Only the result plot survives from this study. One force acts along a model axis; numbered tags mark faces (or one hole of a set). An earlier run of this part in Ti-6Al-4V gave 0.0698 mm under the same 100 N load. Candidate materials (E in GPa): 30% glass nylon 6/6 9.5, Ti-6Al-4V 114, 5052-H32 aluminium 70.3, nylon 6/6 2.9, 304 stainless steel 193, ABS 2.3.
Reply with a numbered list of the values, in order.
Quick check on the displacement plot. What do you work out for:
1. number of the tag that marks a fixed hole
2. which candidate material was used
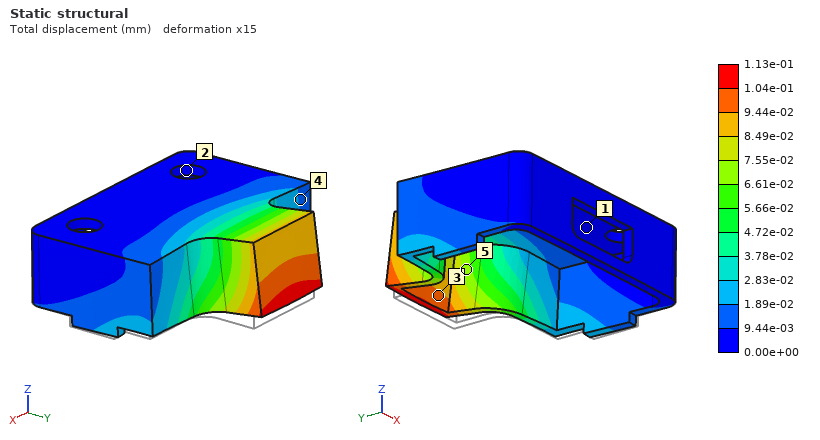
1. 2
2. 5052-H32 aluminium
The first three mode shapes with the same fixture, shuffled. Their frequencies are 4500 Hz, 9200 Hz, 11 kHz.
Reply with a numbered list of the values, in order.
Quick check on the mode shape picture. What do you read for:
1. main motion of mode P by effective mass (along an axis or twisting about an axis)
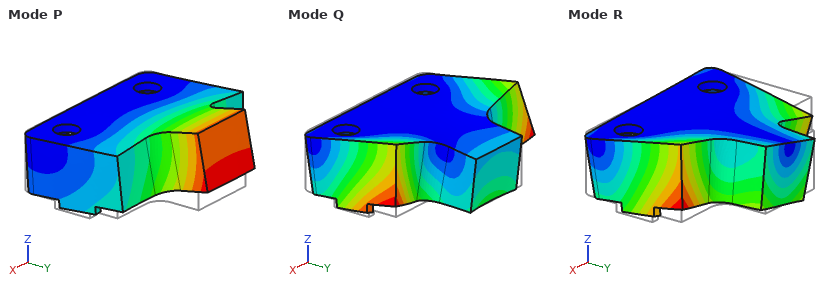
1. along Z
